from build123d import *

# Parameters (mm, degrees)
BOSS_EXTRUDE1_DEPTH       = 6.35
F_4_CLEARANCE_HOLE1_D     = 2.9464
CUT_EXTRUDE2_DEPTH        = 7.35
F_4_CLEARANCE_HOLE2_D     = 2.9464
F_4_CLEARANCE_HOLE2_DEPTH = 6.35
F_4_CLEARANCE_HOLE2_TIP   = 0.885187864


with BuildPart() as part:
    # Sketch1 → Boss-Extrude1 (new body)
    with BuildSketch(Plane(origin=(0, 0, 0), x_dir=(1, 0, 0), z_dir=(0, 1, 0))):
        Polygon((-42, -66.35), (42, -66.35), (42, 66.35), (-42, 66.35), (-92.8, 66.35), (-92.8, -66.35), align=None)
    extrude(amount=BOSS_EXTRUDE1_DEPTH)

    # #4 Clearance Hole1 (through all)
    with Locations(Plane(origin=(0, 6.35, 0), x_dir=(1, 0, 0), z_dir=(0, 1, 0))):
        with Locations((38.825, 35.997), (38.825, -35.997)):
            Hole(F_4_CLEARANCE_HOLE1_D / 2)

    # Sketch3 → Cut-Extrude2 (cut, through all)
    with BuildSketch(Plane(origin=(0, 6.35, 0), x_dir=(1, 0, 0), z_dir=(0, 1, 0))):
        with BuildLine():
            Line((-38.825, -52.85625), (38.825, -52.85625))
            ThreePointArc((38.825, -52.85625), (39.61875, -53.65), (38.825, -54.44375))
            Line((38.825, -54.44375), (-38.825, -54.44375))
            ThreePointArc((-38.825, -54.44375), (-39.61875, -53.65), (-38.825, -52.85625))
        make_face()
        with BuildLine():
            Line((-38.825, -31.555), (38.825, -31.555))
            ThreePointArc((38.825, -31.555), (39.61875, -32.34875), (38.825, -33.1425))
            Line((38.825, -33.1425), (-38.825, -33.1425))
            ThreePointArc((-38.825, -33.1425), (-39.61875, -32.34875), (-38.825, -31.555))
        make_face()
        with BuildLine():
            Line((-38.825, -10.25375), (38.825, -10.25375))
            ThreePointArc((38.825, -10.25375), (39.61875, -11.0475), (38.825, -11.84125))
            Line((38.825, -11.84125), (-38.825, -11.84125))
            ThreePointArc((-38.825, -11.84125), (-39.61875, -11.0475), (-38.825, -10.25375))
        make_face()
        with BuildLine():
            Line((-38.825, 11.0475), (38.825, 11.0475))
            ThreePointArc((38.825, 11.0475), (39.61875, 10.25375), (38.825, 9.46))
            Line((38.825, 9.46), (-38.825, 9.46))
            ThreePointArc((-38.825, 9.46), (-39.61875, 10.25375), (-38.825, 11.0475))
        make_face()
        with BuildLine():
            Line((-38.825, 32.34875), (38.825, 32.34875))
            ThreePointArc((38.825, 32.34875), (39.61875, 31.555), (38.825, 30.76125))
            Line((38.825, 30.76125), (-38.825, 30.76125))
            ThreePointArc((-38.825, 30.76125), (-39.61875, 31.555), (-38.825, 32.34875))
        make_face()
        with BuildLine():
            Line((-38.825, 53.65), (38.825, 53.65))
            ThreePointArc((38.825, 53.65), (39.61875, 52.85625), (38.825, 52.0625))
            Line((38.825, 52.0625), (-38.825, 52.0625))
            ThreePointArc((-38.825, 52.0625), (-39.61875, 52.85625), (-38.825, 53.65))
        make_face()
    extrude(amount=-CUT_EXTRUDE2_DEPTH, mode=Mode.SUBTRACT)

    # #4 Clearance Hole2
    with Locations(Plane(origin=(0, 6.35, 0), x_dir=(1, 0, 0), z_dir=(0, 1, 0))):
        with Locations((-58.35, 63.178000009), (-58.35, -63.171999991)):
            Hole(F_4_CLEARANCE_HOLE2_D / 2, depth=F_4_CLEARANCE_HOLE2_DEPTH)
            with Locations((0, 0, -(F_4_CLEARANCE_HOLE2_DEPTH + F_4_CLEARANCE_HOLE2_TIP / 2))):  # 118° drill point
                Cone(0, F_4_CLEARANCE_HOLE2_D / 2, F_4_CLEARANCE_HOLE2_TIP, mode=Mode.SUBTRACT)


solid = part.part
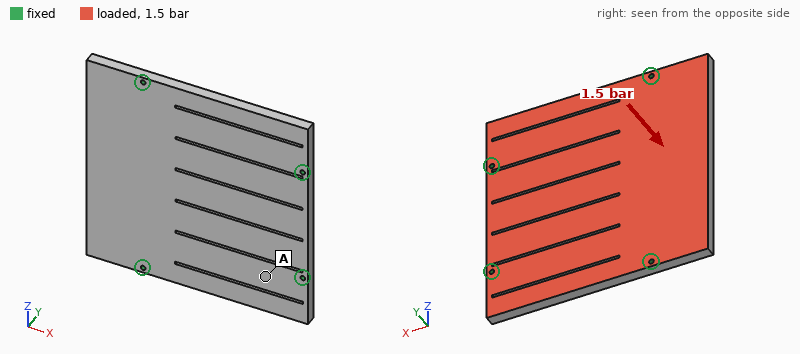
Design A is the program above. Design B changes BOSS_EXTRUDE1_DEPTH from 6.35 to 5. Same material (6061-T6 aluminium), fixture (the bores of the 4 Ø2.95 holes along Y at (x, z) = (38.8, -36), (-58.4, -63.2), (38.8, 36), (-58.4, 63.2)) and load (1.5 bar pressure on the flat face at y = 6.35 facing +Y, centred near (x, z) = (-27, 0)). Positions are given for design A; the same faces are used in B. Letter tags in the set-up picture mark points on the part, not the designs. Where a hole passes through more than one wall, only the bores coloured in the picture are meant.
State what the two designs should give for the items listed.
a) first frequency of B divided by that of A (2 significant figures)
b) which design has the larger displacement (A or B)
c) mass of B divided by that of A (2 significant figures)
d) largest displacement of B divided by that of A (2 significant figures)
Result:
0.81
B
0.79
1.9
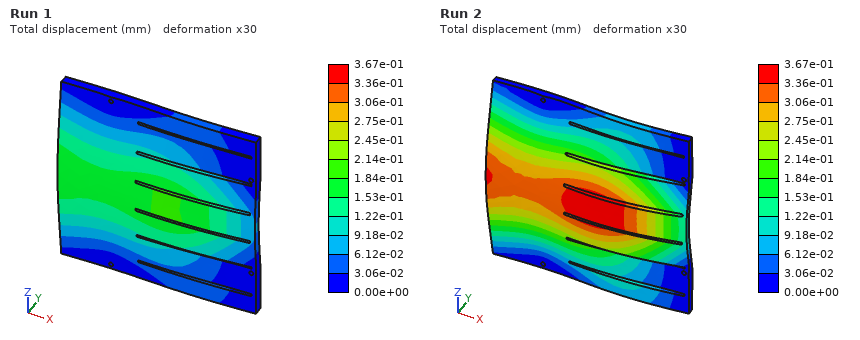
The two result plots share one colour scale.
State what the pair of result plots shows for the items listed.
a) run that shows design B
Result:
Run 2
